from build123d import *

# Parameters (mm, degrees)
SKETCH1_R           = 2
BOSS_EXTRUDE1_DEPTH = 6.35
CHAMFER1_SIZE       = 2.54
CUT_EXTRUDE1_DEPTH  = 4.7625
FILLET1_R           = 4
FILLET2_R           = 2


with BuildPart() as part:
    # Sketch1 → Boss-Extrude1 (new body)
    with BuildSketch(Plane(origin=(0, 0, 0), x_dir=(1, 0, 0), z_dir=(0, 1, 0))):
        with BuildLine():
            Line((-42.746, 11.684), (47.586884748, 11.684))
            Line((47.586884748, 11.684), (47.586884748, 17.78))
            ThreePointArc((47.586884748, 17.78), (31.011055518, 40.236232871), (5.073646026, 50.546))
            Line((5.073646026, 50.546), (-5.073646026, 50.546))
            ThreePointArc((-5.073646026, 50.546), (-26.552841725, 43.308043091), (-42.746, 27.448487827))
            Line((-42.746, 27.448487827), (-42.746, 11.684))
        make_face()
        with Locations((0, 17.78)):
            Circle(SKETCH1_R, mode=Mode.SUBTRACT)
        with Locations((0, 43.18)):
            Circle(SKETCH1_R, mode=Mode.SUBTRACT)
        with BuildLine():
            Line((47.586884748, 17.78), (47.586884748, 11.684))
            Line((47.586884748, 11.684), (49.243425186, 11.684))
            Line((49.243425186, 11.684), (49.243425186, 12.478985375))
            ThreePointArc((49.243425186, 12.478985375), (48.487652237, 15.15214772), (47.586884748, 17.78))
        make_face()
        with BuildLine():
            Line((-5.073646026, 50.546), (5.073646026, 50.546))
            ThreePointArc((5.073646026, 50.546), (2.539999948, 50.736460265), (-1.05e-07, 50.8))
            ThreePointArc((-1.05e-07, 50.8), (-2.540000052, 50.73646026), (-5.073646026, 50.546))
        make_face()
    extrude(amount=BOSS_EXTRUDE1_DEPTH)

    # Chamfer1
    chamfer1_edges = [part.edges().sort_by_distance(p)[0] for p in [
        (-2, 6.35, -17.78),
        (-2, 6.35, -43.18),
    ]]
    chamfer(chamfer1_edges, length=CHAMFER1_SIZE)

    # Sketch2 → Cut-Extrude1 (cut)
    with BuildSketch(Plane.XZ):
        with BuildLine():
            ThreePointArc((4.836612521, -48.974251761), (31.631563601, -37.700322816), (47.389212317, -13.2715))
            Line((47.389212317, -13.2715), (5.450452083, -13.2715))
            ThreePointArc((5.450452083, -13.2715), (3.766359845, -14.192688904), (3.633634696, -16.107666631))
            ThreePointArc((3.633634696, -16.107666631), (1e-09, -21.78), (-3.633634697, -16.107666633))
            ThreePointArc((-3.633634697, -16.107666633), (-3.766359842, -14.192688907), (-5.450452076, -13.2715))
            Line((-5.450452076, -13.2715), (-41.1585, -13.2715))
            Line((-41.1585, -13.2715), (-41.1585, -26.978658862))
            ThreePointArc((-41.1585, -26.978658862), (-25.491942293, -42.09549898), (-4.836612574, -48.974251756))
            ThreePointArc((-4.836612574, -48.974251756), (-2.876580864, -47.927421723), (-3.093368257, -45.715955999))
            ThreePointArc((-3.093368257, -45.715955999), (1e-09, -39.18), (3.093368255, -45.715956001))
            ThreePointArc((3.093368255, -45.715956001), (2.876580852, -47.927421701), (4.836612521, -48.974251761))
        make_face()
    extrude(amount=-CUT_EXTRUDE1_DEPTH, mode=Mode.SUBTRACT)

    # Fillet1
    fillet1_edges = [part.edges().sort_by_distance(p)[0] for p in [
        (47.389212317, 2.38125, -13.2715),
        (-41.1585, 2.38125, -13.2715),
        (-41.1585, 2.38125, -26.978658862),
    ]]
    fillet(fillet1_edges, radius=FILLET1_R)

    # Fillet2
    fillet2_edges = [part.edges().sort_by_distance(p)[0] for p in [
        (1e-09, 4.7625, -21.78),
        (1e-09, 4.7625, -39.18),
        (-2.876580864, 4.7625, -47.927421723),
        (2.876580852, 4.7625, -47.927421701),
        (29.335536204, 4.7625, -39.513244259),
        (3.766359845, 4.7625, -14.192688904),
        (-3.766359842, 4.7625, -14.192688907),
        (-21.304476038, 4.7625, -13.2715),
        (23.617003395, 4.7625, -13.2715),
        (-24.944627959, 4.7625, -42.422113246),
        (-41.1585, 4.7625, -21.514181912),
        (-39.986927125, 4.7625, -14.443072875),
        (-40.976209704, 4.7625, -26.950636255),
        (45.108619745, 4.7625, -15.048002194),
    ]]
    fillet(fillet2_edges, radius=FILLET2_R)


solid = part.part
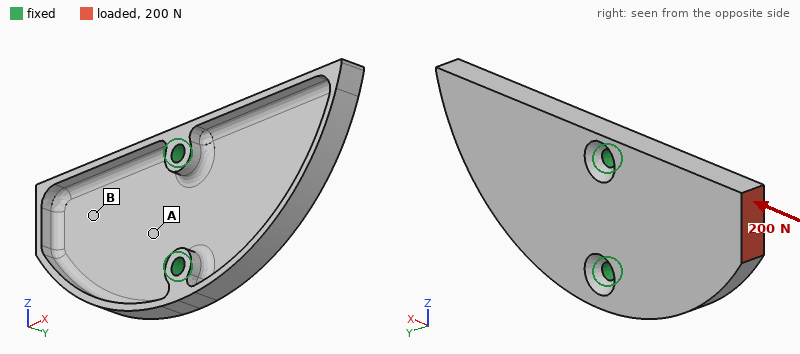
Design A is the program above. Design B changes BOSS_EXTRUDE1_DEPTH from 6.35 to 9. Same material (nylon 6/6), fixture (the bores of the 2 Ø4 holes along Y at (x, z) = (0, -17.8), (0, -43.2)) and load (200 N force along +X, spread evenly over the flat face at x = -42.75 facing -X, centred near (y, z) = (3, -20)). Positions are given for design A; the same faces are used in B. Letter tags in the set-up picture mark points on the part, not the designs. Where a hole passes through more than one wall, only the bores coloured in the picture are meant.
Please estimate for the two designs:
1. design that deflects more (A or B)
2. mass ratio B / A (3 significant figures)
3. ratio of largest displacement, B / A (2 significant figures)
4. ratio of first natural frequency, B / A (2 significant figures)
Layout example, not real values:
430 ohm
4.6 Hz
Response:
A
2.10
0.31
1.4
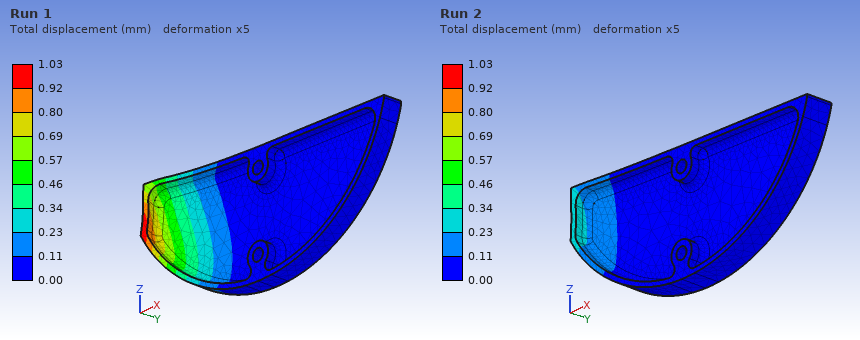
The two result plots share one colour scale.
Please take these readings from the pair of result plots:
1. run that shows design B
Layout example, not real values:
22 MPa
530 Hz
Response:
Run 2
